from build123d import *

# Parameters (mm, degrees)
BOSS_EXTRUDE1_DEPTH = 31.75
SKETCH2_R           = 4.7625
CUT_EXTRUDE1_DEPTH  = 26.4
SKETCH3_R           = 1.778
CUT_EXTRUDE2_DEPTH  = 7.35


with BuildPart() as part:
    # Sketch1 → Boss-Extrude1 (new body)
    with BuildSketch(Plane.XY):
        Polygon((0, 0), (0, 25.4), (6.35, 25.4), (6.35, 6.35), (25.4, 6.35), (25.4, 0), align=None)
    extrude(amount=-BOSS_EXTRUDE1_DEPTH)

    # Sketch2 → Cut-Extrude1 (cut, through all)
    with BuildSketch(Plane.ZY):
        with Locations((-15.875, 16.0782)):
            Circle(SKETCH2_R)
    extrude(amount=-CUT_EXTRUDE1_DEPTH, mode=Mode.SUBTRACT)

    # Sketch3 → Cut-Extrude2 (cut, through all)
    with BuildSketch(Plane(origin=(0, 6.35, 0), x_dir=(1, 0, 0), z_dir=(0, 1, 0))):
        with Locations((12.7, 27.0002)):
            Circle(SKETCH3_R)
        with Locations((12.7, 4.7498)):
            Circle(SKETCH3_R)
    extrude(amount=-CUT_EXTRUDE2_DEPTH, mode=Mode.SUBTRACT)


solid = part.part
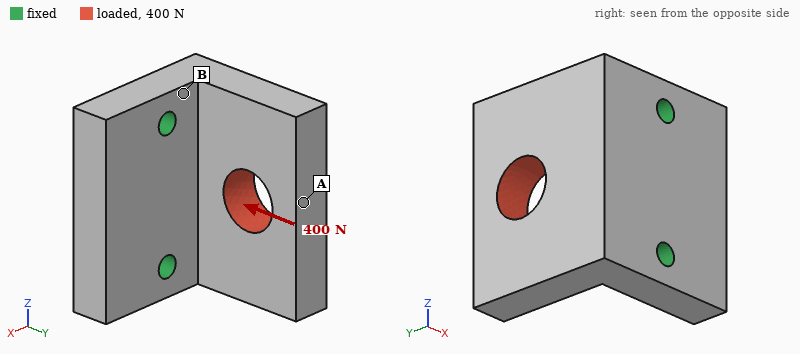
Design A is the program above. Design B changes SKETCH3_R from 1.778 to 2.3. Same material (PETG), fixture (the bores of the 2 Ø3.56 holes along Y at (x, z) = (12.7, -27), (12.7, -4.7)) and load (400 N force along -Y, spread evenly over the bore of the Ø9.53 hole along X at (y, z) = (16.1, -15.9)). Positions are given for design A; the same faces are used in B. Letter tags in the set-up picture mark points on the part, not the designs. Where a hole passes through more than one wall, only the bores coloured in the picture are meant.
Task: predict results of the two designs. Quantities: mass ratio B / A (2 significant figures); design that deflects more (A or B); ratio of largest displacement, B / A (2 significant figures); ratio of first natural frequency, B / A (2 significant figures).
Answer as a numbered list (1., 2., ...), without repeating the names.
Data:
1. 0.99
2. A
3. 0.85
4. 1.0
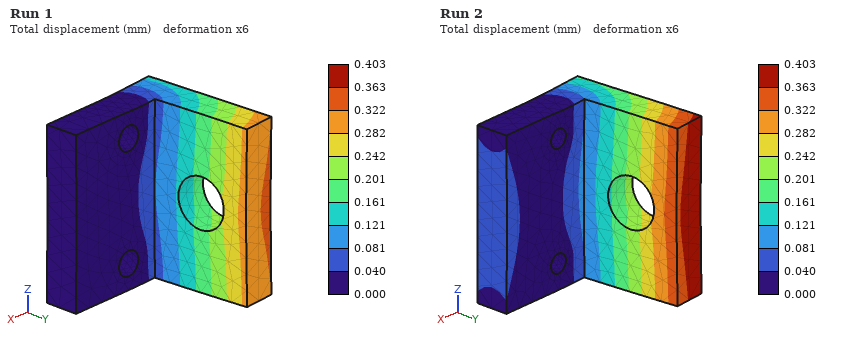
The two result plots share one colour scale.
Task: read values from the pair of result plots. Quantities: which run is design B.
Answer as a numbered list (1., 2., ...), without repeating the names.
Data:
1. Run 1
